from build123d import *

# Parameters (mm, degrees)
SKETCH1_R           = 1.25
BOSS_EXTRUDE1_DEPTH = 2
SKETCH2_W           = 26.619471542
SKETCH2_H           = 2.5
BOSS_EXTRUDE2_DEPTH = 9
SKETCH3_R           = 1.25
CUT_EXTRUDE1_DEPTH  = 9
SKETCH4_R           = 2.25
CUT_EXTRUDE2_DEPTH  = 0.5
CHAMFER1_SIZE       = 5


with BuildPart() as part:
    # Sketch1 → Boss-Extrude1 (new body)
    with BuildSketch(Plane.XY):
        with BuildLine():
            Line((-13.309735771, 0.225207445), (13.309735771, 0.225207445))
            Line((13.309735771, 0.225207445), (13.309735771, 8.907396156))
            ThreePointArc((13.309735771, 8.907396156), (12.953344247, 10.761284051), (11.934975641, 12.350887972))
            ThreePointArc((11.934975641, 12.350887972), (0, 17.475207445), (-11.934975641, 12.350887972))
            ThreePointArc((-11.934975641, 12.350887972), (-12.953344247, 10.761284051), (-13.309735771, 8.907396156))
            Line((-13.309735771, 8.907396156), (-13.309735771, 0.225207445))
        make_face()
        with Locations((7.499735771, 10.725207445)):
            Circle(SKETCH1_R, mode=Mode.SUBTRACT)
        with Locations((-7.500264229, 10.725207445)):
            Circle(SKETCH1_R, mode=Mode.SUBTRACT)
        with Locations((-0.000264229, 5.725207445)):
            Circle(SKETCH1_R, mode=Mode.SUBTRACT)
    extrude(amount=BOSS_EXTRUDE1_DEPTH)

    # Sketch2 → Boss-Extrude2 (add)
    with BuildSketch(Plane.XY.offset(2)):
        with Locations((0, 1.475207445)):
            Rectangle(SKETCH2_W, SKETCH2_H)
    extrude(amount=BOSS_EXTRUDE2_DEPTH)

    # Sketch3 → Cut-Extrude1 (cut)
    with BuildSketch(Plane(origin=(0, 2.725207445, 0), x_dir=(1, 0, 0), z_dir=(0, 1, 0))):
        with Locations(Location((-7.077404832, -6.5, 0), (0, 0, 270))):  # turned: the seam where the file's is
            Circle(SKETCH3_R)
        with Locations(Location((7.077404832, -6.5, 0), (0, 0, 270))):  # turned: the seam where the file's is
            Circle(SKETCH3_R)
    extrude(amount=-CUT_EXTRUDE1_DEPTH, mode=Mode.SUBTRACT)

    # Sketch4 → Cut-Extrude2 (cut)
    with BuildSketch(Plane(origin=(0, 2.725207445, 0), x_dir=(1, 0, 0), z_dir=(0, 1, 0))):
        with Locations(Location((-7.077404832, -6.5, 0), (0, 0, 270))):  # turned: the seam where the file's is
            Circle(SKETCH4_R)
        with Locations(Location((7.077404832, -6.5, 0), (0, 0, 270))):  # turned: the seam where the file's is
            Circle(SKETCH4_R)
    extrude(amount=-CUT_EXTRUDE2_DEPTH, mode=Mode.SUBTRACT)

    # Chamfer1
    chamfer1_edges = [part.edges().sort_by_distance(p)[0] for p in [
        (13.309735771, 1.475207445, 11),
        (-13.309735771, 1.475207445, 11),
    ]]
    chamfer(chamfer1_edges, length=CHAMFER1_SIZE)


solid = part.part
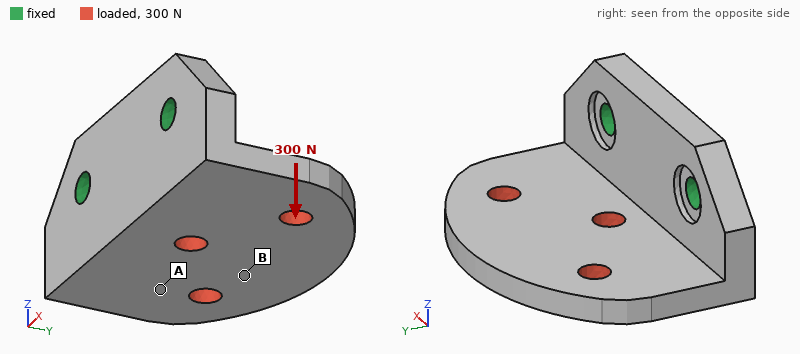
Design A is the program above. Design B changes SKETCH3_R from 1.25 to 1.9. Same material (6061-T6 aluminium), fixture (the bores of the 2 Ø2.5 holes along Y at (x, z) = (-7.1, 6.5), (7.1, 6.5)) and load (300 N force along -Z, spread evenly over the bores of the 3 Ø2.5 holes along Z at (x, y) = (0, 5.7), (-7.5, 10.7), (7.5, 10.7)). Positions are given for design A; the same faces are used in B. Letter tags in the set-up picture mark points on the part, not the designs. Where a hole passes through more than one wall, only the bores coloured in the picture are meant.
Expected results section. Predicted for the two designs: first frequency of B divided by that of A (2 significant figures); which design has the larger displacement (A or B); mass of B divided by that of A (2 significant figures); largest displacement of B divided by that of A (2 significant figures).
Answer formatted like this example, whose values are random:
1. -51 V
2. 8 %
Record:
1. 1.1
2. A
3. 0.98
4. 0.86
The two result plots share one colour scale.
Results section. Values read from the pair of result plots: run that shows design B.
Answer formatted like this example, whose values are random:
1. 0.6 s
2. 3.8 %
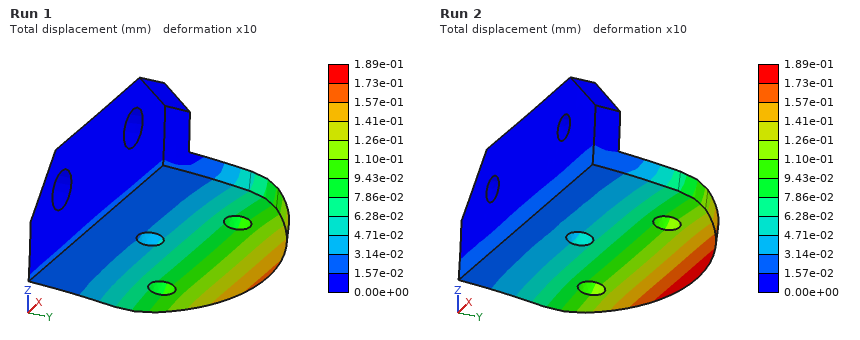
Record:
1. Run 1
